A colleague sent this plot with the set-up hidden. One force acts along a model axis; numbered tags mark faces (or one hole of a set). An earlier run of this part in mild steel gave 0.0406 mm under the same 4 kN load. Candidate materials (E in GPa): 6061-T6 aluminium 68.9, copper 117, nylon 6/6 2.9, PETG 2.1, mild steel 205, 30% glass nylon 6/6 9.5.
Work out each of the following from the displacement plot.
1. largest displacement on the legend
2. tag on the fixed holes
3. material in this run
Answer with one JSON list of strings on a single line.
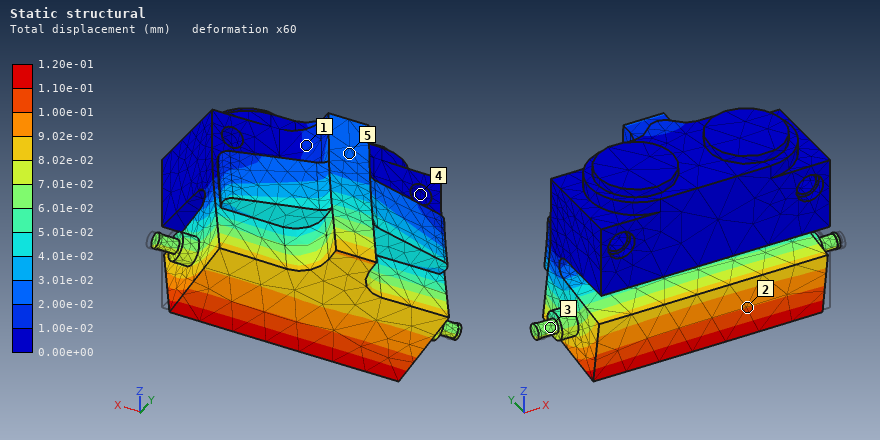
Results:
["1.20e-01 mm", "4", "6061-T6 aluminium"]
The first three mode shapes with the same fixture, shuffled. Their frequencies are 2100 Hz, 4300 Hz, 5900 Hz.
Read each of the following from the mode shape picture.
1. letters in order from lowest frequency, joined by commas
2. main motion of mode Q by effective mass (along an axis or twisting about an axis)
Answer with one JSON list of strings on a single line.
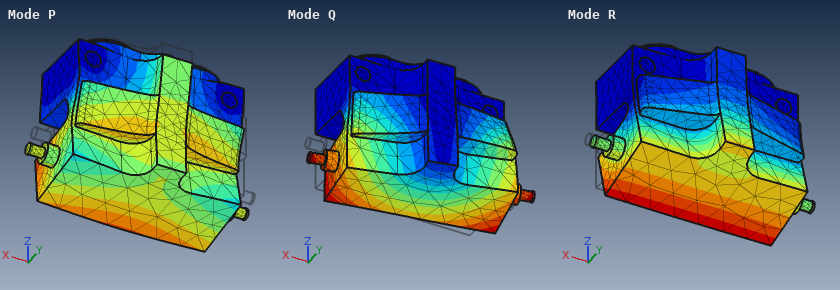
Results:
["R, Q, P", "along X"]
